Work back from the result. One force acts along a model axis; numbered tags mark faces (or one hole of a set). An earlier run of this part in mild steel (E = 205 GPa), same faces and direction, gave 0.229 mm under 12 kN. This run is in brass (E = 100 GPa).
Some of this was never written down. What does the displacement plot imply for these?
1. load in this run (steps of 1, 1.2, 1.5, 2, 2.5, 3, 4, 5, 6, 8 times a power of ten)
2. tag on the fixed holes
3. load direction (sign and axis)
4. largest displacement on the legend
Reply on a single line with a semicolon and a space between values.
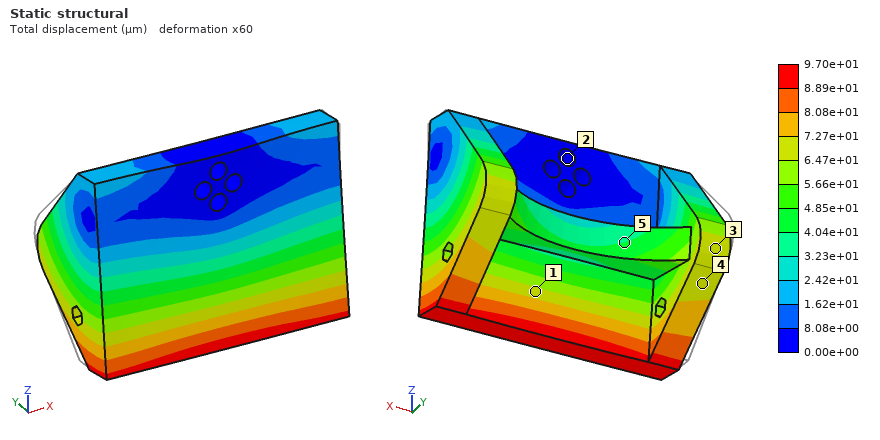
2.5 kN; 2; -Y; 9.70e+01 µm
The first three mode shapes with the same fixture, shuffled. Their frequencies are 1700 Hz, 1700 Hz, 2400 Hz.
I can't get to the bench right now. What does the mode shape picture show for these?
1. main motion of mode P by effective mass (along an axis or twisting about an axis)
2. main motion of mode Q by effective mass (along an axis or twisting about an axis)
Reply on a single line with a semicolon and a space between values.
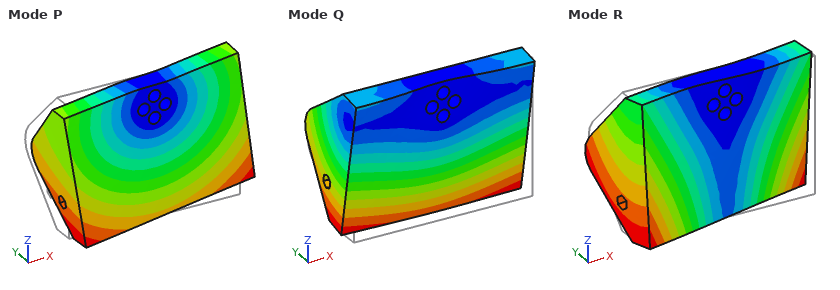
along X; along Y
